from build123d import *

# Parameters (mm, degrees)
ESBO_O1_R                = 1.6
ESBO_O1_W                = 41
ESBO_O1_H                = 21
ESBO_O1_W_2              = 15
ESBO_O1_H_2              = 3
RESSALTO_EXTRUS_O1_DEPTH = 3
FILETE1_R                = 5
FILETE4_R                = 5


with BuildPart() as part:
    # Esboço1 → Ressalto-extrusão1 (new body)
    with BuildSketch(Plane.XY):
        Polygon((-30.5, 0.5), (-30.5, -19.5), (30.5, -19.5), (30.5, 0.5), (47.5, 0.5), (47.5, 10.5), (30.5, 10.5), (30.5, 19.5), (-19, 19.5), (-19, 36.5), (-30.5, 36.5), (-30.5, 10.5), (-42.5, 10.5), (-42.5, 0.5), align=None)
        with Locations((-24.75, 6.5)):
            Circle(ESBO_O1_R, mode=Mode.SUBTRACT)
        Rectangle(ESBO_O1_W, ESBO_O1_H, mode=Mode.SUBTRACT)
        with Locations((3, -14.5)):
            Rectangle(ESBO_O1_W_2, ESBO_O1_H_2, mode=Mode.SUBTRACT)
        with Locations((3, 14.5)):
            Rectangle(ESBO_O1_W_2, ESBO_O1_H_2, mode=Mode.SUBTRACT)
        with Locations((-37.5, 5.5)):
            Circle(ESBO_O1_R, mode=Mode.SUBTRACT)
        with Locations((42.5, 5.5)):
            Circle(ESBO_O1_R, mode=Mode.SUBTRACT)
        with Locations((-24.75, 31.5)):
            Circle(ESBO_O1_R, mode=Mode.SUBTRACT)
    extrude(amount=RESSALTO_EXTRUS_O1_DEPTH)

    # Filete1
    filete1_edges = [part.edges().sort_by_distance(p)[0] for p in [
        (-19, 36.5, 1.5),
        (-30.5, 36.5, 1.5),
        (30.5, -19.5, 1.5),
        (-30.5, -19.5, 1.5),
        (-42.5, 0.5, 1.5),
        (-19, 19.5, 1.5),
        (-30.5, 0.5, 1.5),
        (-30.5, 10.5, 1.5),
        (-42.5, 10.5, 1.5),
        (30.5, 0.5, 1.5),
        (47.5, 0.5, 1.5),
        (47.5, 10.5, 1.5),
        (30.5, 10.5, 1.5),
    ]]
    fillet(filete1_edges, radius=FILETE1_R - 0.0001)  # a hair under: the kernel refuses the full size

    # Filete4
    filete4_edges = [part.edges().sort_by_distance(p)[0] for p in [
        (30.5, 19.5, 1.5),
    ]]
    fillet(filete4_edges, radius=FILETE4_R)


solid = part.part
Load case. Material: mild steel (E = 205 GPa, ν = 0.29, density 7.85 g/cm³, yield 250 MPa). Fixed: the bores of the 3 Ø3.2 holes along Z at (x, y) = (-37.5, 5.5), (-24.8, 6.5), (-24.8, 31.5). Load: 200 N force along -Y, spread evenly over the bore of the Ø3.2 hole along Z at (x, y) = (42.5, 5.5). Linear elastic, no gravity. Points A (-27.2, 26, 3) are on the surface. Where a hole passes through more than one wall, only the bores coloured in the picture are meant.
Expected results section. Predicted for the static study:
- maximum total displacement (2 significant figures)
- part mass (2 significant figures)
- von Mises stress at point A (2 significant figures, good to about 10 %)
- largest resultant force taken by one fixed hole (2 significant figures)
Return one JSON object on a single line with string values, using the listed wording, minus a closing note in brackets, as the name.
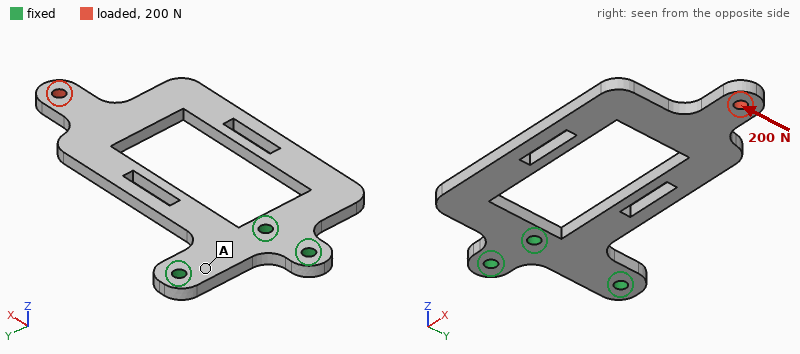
{"maximum total displacement": "98 µm", "part mass": "44 g", "von Mises stress at point A": "15 MPa", "largest resultant force taken by one fixed hole": "540 N"}
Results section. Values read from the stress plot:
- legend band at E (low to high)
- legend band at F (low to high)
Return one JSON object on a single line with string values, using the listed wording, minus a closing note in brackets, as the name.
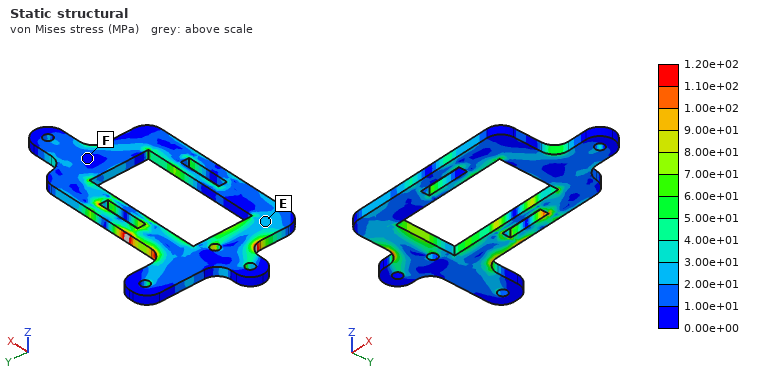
{"legend band at E": "2.00e+01 to 3.00e+01 MPa", "legend band at F": "0.00e+00 to 1.00e+01 MPa"}
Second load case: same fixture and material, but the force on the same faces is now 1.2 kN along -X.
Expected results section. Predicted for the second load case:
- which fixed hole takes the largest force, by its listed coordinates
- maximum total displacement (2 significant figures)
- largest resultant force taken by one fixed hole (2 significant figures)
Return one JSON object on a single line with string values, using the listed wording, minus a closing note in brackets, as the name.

{"which fixed hole takes the largest force, by its listed coordinates": "(-24.8, 6.5)", "maximum total displacement": "42 µm", "largest resultant force taken by one fixed hole": "680 N"}
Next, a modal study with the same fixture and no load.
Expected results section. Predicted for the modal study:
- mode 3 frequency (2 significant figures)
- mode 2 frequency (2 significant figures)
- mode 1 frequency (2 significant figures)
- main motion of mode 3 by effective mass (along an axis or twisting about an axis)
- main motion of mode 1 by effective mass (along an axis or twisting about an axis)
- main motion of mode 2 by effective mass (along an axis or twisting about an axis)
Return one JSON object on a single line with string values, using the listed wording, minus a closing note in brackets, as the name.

{"mode 3 frequency": "2000 Hz", "mode 2 frequency": "1400 Hz", "mode 1 frequency": "440 Hz", "main motion of mode 3 by effective mass": "along Y", "main motion of mode 1 by effective mass": "along Z", "main motion of mode 2 by effective mass": "twisting about X"}
